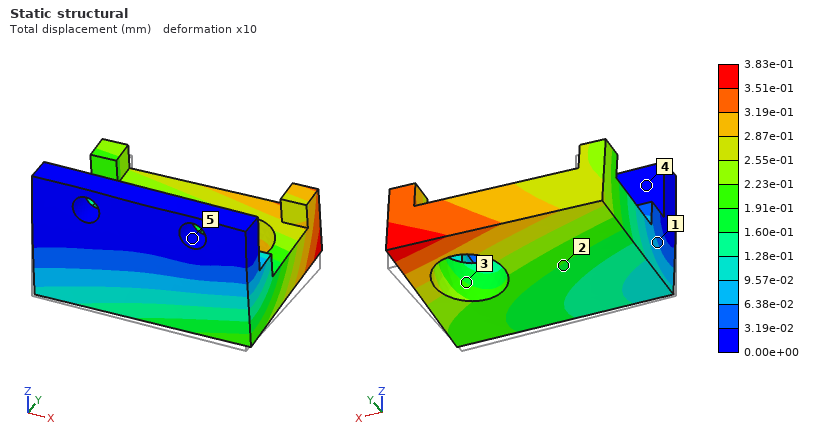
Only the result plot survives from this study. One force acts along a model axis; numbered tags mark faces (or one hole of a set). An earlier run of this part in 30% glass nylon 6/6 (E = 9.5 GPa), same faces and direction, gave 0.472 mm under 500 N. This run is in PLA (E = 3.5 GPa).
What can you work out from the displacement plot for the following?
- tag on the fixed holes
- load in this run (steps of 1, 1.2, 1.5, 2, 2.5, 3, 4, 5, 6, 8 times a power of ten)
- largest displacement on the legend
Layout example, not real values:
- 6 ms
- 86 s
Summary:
- 5
- 150 N
- 3.83e-01 mm
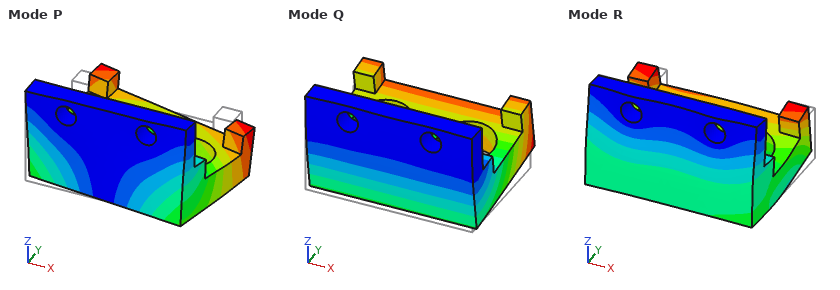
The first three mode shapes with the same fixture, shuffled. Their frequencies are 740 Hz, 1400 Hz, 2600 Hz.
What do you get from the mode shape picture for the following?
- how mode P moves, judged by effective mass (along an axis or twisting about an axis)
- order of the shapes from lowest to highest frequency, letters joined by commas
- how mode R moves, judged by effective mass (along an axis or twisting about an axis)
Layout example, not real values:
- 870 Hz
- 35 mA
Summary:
- along X
- Q, P, R
- along Y
